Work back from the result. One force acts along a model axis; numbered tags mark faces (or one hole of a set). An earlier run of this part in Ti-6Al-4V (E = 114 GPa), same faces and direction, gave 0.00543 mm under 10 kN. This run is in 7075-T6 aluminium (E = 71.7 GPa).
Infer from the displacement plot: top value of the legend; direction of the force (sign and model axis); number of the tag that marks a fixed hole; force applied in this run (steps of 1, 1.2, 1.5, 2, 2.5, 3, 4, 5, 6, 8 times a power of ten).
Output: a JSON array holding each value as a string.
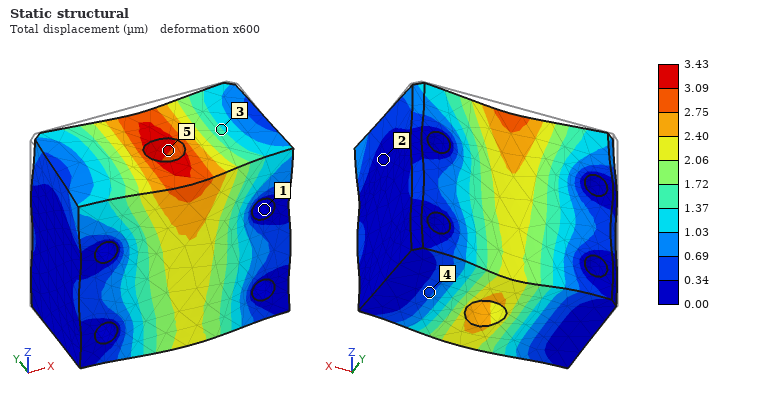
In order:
["3.43 µm", "-Y", "1", "4 kN"]
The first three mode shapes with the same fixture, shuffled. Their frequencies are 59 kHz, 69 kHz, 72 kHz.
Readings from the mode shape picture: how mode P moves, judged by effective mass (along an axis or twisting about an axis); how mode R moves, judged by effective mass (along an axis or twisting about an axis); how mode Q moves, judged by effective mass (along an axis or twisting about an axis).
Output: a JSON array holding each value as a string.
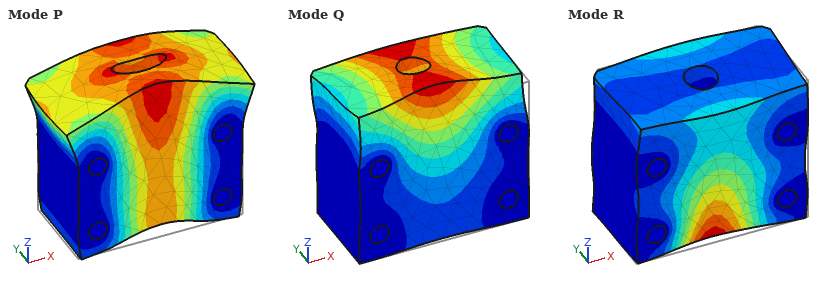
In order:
["along Z", "along Y", "along Y"]
